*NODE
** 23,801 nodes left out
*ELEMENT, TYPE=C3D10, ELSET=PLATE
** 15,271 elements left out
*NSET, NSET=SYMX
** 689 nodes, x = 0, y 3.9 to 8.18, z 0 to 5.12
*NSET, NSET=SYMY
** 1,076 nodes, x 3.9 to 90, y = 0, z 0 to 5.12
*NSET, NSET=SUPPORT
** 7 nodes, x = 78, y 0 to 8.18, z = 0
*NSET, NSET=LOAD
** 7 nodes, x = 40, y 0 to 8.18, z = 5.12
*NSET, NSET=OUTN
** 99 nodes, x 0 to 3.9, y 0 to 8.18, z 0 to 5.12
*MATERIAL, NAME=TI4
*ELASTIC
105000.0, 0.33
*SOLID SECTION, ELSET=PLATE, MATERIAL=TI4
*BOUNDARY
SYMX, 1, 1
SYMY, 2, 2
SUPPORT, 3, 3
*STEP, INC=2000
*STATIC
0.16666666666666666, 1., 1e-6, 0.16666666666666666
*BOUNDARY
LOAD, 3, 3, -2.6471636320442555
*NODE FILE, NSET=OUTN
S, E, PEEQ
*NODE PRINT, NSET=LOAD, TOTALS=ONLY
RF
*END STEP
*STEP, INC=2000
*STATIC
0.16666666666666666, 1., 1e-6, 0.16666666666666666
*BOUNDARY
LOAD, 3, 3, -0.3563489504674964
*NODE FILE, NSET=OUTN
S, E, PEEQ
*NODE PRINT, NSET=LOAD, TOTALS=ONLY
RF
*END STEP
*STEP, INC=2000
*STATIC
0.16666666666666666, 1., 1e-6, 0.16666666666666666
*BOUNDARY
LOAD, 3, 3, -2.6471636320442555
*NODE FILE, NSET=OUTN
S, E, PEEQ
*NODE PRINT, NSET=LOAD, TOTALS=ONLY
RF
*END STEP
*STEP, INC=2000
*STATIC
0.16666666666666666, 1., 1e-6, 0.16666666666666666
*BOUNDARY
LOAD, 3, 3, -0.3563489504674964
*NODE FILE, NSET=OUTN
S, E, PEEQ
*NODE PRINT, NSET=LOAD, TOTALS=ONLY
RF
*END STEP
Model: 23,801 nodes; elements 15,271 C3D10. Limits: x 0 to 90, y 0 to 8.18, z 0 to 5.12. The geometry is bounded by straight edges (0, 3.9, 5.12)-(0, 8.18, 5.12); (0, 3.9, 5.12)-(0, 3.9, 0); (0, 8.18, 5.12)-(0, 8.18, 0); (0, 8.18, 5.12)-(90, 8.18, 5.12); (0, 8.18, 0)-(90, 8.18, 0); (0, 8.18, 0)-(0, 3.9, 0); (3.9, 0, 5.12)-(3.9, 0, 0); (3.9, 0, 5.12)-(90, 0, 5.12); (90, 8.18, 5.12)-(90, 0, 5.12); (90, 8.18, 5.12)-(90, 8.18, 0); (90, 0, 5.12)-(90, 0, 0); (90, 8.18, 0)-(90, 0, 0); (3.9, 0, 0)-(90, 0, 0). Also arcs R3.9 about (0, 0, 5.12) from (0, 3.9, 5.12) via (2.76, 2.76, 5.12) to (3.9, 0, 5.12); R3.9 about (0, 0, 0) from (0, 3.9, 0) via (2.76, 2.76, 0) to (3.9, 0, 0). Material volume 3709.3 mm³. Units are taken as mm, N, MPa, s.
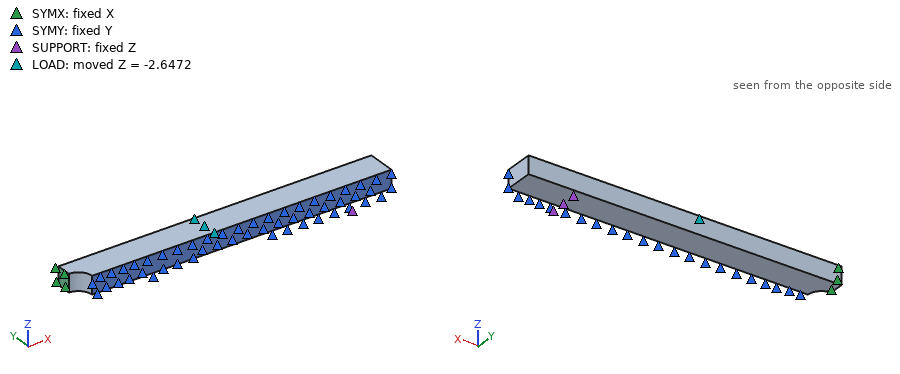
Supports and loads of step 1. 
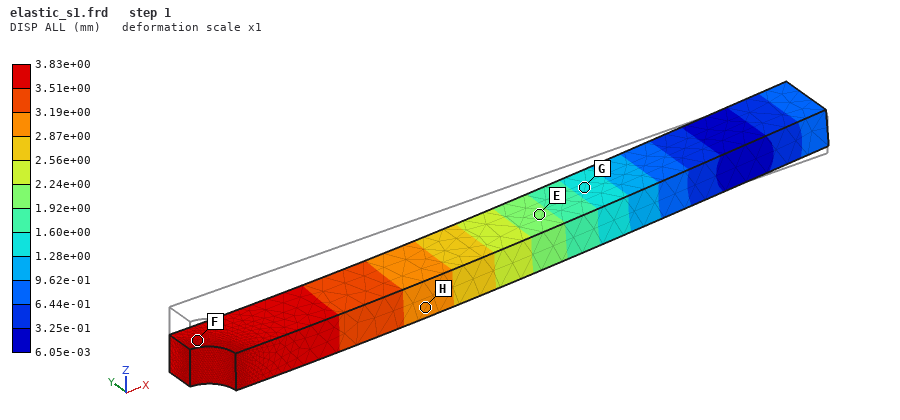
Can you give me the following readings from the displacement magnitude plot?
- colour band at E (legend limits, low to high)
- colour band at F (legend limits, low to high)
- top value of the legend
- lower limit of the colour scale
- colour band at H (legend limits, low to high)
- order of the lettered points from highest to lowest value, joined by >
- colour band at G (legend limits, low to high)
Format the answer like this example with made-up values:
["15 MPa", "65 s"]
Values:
["1.92e+00 to 2.24e+00 mm", "3.51e+00 to 3.83e+00 mm", "3.83e+00 mm", "6.05e-03 mm", "2.87e+00 to 3.19e+00 mm", "F > H > E > G", "1.28e+00 to 1.60e+00 mm"]
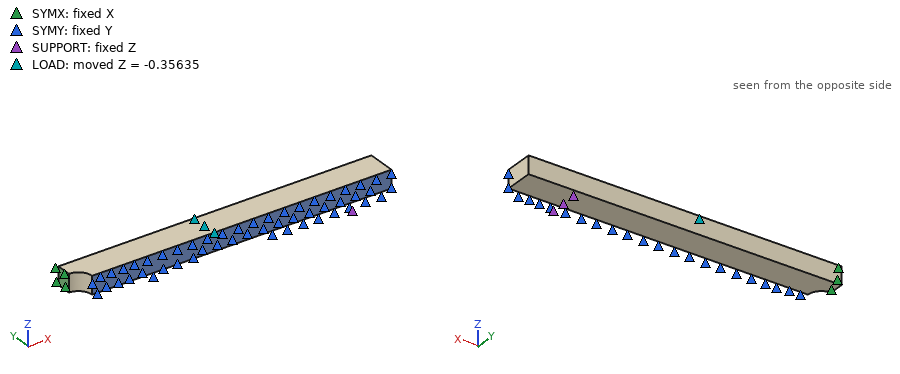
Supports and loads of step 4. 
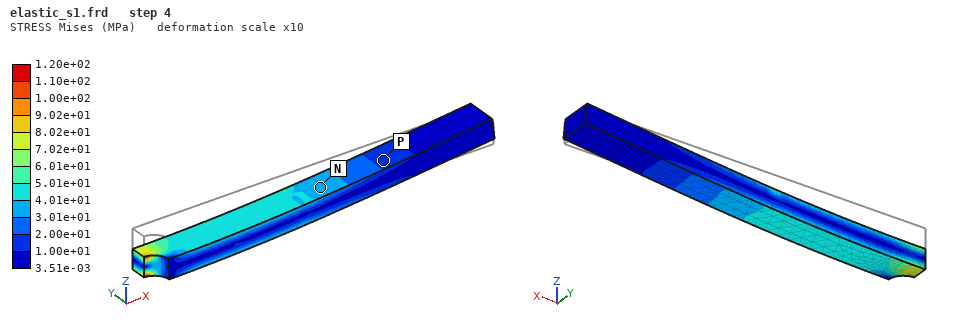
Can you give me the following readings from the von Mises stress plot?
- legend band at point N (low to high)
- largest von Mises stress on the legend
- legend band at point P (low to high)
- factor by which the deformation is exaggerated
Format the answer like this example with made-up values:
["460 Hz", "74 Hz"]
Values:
["3.01e+01 to 4.01e+01 MPa", "1.20e+02 MPa", "1.00e+01 to 2.00e+01 MPa", "10"]
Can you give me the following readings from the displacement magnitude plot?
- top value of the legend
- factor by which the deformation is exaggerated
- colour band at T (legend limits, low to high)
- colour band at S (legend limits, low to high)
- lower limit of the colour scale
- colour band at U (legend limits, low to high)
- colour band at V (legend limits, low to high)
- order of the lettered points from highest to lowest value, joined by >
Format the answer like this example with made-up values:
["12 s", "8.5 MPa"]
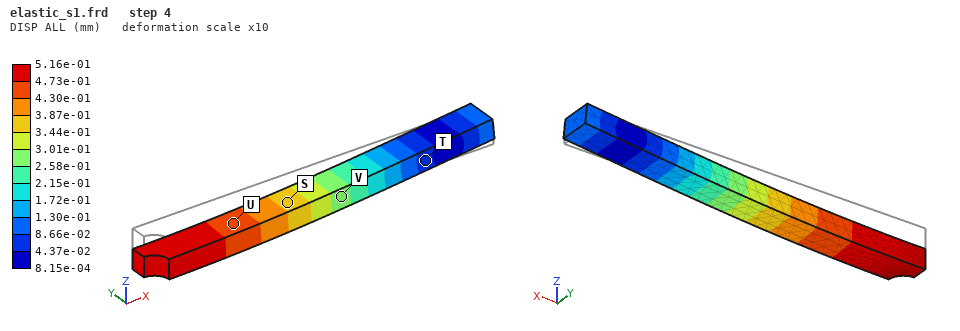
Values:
["5.16e-01 mm", "10", "4.37e-02 to 8.66e-02 mm", "3.44e-01 to 3.87e-01 mm", "8.15e-04 mm", "4.30e-01 to 4.73e-01 mm", "2.58e-01 to 3.01e-01 mm", "U > S > V > T"]
